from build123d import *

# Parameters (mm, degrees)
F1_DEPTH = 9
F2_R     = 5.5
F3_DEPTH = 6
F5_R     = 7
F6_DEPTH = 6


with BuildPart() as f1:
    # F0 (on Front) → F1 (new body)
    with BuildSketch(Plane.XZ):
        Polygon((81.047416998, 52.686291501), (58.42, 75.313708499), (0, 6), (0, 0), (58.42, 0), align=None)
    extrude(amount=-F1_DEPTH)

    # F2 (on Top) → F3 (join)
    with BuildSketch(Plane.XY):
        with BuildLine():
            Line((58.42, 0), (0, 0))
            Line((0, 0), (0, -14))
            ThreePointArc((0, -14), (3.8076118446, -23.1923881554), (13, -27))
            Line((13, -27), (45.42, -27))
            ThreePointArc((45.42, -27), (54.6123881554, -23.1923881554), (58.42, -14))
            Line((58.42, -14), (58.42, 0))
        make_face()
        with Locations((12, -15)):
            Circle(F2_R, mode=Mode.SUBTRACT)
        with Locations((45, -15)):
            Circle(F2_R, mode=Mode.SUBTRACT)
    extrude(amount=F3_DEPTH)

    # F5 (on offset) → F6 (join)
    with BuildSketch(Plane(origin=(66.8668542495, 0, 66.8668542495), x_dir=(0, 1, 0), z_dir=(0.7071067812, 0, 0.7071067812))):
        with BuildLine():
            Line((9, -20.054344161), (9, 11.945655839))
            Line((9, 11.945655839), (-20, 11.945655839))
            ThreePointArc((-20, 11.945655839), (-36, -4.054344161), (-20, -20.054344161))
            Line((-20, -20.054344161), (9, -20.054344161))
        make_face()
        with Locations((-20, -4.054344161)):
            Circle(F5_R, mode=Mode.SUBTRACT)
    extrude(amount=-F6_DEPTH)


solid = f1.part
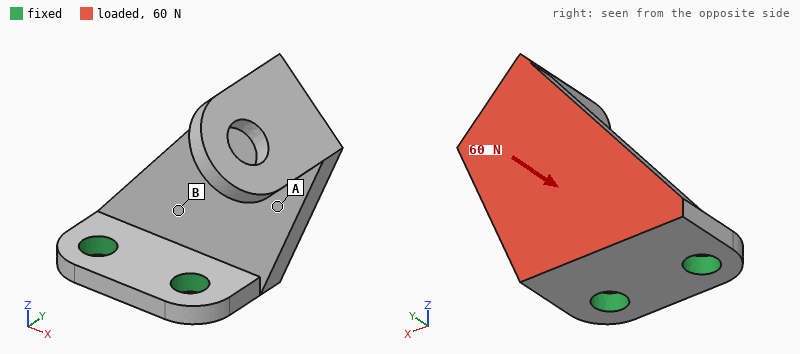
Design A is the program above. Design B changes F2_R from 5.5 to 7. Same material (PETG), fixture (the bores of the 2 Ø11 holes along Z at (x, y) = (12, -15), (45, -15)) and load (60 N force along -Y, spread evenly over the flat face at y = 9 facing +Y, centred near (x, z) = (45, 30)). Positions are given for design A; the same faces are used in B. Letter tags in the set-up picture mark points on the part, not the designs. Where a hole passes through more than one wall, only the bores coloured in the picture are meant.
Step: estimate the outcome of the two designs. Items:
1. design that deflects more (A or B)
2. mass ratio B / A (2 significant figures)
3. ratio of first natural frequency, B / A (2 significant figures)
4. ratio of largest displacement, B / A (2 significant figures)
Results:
A
0.98
1.0
0.92
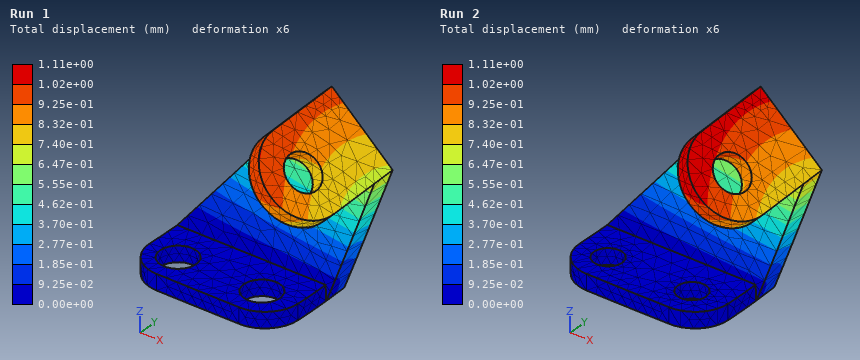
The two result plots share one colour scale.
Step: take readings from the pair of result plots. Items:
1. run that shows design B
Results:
Run 1
